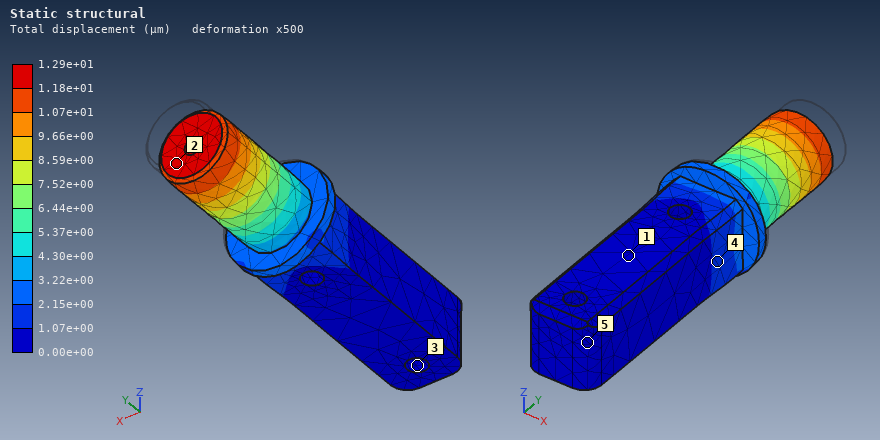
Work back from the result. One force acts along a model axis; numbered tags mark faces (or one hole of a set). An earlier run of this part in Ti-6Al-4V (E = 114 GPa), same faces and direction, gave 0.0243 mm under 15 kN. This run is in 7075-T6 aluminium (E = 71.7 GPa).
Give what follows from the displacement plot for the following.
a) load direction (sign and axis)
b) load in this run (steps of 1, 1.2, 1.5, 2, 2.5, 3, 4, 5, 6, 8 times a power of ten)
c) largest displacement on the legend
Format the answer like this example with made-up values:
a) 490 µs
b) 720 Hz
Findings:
a) -Y
b) 5 kN
c) 1.29e+01 µm
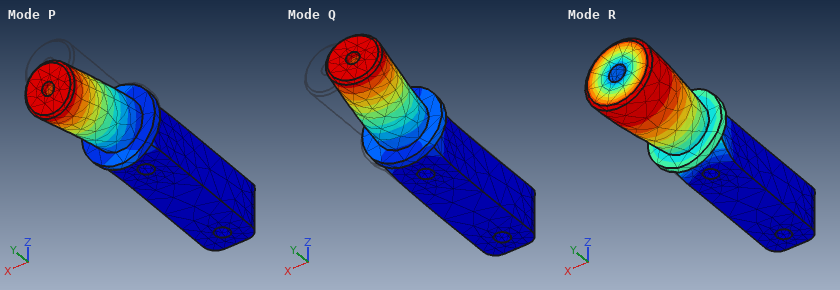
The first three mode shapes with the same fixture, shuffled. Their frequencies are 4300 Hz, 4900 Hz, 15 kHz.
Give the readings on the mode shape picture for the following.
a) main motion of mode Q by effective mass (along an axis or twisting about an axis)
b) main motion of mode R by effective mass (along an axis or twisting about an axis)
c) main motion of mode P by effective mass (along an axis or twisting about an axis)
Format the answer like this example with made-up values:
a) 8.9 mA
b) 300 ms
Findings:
a) along X
b) twisting about Y
c) along Z
